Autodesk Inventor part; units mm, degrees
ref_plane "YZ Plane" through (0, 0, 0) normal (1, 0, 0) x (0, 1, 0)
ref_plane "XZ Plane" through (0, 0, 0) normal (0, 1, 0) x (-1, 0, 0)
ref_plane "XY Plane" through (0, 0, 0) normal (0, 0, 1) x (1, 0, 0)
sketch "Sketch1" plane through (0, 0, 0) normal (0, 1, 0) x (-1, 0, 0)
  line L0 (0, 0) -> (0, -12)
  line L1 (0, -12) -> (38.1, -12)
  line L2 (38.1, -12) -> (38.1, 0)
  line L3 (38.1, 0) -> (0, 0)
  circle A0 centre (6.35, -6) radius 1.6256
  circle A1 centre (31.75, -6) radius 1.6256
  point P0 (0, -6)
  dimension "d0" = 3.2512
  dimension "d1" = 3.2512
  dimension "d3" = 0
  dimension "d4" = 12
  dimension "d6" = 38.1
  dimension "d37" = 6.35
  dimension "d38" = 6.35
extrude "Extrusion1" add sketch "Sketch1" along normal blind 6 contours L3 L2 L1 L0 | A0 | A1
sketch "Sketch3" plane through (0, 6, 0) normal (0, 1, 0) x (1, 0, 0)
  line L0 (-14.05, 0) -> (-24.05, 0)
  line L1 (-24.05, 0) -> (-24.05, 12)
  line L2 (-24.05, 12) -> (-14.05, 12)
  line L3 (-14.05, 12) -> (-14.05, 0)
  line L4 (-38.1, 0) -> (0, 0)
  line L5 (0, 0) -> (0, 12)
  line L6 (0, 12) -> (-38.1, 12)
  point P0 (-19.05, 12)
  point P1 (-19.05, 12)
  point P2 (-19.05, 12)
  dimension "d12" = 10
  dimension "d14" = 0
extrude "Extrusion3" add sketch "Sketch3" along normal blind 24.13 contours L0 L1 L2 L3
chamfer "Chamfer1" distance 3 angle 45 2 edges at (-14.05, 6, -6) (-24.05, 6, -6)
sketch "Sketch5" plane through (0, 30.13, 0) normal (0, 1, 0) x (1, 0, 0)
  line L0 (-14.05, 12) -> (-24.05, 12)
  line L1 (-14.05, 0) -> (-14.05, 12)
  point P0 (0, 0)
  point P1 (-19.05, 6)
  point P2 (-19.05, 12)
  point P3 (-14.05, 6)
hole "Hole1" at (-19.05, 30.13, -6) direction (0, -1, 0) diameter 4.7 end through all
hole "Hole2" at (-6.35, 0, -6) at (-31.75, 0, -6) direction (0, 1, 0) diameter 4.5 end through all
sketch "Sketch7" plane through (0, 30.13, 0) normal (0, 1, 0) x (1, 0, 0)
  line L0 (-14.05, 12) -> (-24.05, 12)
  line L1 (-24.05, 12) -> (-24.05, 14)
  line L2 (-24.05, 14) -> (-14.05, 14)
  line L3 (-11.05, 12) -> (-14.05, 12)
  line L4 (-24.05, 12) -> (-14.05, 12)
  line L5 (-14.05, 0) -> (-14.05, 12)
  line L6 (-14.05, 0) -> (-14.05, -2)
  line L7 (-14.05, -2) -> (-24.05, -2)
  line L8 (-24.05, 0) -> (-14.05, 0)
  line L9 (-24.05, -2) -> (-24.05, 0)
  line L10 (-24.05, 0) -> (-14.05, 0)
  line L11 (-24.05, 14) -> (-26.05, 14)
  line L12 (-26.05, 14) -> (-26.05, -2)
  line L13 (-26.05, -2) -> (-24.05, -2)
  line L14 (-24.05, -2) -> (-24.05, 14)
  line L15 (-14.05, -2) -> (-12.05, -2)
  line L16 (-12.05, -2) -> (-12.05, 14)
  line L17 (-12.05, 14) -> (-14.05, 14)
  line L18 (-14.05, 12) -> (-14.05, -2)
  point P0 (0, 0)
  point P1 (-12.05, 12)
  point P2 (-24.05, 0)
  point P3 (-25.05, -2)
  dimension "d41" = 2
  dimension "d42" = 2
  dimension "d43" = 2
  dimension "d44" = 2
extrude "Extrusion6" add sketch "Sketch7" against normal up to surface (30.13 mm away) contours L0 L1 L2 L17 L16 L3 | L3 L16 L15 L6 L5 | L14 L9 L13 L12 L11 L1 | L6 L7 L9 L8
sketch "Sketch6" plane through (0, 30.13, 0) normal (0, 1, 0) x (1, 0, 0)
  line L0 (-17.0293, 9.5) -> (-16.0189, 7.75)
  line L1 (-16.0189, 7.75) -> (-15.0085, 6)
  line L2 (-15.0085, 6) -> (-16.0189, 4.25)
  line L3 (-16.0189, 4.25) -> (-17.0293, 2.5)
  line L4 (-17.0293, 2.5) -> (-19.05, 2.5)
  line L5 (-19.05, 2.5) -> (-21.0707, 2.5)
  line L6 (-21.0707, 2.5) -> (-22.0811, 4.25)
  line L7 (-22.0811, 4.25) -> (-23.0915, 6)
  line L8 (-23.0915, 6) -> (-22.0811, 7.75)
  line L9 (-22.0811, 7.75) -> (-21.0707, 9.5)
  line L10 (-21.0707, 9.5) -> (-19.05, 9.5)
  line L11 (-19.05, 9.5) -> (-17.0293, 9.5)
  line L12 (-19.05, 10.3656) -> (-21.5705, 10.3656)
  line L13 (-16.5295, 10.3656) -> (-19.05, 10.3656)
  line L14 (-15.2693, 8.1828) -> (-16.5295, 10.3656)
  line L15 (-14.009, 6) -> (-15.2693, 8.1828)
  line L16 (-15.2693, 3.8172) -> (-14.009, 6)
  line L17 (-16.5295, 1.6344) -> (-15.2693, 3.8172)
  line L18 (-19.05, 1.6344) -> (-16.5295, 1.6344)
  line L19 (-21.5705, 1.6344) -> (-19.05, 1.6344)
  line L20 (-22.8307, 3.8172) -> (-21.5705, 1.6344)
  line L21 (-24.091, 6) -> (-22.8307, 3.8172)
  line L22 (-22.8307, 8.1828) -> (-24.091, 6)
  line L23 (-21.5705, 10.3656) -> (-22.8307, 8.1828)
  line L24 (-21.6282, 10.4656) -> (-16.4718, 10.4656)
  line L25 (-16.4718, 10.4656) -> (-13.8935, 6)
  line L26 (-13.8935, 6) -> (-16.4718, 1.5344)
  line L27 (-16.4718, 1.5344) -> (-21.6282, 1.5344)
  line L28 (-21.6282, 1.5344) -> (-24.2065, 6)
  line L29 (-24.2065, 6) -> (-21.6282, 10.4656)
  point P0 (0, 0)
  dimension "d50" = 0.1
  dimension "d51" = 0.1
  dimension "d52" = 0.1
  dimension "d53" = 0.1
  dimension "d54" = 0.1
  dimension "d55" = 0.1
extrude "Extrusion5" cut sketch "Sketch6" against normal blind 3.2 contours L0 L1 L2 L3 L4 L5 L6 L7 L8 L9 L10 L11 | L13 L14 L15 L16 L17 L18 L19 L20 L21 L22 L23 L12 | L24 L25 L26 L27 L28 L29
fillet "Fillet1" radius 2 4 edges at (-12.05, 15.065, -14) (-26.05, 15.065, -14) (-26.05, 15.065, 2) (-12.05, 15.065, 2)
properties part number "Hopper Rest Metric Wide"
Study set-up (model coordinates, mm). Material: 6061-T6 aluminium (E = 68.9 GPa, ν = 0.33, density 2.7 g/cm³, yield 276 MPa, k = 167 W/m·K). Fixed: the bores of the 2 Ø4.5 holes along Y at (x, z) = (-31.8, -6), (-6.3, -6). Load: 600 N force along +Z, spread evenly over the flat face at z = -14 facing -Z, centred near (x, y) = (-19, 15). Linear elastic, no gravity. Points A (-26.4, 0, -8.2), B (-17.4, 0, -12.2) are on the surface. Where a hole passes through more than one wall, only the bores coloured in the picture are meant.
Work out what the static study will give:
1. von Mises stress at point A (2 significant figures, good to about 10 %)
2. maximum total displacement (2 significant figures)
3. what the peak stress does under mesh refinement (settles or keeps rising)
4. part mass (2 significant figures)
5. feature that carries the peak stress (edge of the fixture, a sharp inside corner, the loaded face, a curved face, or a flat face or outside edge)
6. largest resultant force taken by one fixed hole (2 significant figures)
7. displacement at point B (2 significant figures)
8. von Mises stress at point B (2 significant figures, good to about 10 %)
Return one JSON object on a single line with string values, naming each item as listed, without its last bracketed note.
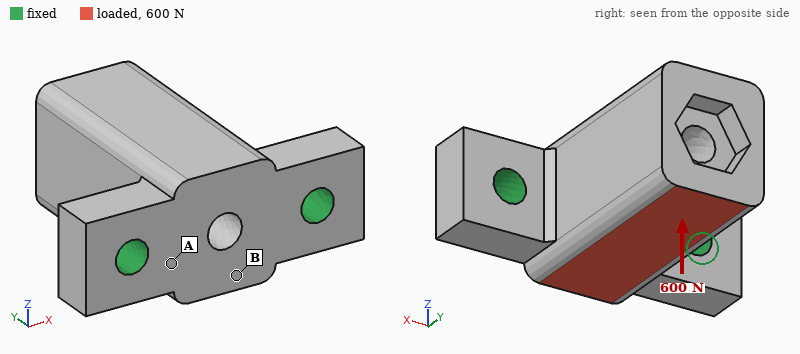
{"von Mises stress at point A": "22 MPa", "maximum total displacement": "40 µm", "what the peak stress does under mesh refinement": "keeps rising", "part mass": "20 g", "feature that carries the peak stress": "edge of the fixture", "largest resultant force taken by one fixed hole": "300 N", "displacement at point B": "7.5 µm", "von Mises stress at point B": "11 MPa"}
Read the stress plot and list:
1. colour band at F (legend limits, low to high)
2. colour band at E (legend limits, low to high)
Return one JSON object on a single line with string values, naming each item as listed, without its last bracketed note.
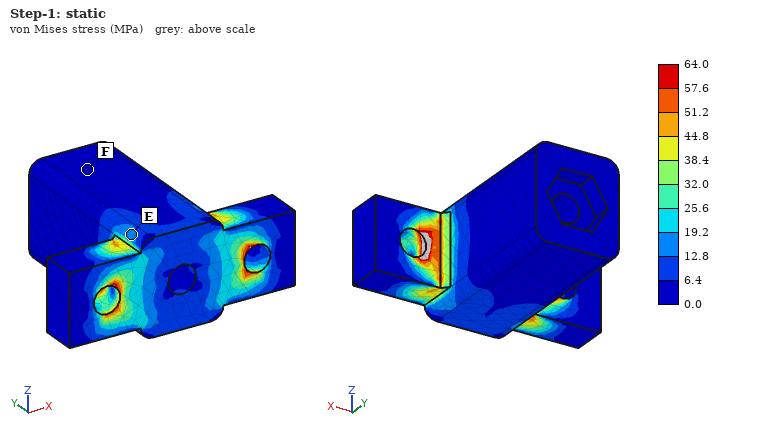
{"colour band at F": "0.0 to 6.4 MPa", "colour band at E": "12.8 to 19.2 MPa"}
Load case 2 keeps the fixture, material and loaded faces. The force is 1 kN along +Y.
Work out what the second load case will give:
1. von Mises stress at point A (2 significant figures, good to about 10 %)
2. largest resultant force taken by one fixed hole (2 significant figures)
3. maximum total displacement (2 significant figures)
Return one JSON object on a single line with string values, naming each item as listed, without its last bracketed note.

{"von Mises stress at point A": "34 MPa", "largest resultant force taken by one fixed hole": "540 N", "maximum total displacement": "45 µm"}
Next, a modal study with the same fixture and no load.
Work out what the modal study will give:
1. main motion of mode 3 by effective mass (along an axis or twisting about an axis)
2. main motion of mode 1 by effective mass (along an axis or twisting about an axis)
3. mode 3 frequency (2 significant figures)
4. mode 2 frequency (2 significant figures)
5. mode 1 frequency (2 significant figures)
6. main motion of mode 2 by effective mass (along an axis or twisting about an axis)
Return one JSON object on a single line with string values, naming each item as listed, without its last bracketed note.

{"main motion of mode 3 by effective mass": "along Y", "main motion of mode 1 by effective mass": "along Z", "mode 3 frequency": "22 kHz", "mode 2 frequency": "12 kHz", "mode 1 frequency": "6000 Hz", "main motion of mode 2 by effective mass": "along X"}
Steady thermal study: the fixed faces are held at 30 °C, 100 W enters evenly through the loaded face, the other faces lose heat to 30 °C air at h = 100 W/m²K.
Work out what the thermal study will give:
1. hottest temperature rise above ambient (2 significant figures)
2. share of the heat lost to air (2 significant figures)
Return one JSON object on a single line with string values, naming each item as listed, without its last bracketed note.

{"hottest temperature rise above ambient": "65 K", "share of the heat lost to air": "9.2 %"}
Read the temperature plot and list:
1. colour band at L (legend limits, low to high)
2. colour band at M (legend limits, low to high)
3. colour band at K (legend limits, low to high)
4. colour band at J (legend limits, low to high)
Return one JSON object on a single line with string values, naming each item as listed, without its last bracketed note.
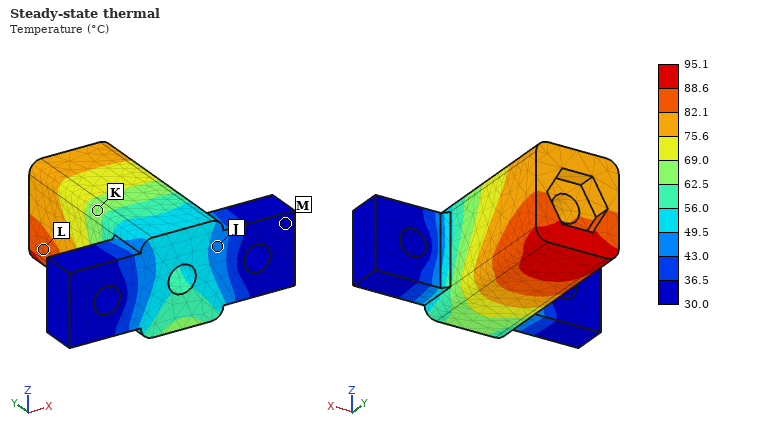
{"colour band at L": "82.1 to 88.6 °C", "colour band at M": "30.0 to 36.5 °C", "colour band at K": "62.5 to 69.0 °C", "colour band at J": "43.0 to 49.5 °C"}
